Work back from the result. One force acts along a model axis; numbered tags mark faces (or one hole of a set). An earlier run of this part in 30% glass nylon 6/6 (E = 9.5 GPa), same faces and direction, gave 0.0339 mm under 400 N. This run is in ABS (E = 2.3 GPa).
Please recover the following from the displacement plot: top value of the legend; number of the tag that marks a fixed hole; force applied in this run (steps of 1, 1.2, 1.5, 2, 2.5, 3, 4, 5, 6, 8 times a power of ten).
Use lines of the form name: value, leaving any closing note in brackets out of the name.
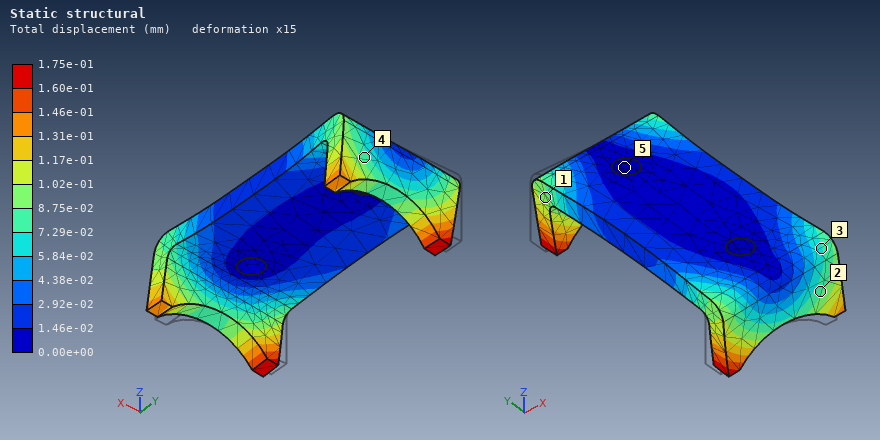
top value of the legend: 1.75e-01 mm
number of the tag that marks a fixed hole: 5
force applied in this run: 500 N
